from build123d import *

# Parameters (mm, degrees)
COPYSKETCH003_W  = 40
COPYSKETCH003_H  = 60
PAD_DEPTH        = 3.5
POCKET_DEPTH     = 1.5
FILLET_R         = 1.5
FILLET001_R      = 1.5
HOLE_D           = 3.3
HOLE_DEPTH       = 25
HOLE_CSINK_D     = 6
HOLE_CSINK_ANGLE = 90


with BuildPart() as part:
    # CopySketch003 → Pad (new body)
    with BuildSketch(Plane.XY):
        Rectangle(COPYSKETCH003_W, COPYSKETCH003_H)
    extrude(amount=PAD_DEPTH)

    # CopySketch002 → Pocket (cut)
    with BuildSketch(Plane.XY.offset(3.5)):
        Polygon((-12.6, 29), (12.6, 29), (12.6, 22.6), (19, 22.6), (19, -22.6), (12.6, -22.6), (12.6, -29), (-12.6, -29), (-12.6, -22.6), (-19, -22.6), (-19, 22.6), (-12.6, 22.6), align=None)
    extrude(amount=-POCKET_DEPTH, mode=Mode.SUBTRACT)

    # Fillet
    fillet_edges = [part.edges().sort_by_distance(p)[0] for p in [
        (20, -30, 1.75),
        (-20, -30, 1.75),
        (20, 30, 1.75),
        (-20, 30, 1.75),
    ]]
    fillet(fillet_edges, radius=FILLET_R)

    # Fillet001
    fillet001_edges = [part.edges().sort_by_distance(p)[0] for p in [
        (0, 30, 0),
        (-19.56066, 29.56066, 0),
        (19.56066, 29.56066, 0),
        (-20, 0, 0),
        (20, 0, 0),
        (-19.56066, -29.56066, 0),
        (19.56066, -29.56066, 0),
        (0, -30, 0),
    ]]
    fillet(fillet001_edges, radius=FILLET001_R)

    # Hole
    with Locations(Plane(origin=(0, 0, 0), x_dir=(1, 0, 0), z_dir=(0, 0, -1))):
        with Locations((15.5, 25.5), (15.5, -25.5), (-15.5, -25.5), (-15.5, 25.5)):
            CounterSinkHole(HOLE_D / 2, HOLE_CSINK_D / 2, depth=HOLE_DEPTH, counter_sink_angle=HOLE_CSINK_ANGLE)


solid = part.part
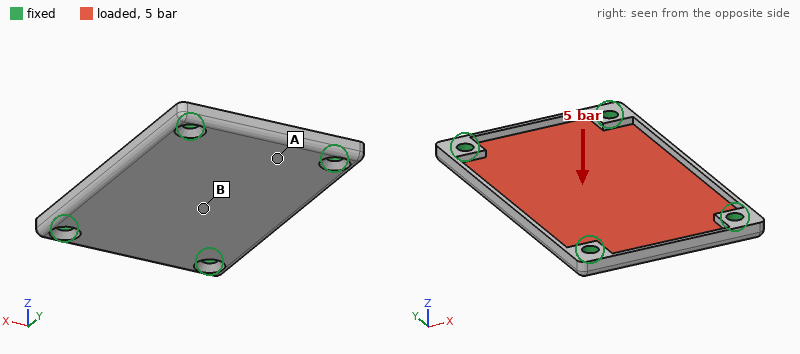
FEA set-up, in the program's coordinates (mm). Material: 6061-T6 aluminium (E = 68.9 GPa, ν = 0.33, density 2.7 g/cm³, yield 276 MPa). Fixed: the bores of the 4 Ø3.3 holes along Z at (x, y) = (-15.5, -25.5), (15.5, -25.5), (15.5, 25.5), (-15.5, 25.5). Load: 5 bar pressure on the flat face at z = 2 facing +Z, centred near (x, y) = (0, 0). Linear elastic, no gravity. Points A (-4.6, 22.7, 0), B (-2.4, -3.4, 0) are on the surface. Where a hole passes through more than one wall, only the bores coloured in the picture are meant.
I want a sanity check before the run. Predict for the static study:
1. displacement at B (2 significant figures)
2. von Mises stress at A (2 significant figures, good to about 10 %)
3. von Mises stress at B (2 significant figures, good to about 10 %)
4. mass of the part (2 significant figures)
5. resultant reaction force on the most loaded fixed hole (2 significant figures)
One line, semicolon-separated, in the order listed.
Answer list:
0.18 mm; 43 MPa; 68 MPa; 14 g; 400 N
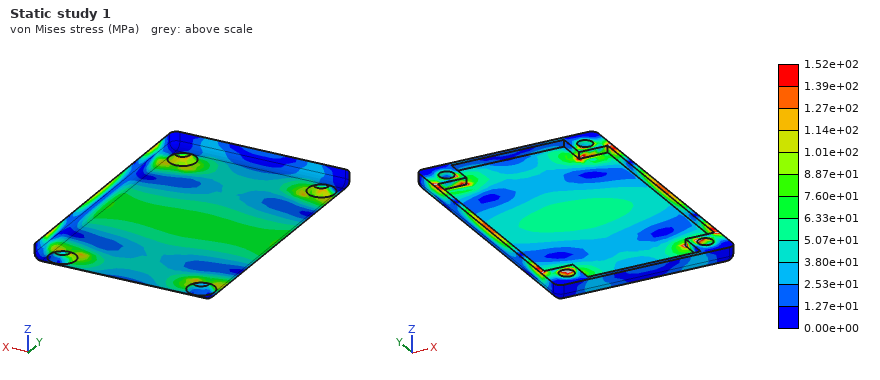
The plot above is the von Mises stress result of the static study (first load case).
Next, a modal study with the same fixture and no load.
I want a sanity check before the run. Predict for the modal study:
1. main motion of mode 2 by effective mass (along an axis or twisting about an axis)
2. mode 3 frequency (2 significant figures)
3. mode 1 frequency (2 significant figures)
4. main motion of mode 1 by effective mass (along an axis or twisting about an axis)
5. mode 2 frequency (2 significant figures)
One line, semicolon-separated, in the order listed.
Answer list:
twisting about Y; 9700 Hz; 4100 Hz; along Z; 6100 Hz
